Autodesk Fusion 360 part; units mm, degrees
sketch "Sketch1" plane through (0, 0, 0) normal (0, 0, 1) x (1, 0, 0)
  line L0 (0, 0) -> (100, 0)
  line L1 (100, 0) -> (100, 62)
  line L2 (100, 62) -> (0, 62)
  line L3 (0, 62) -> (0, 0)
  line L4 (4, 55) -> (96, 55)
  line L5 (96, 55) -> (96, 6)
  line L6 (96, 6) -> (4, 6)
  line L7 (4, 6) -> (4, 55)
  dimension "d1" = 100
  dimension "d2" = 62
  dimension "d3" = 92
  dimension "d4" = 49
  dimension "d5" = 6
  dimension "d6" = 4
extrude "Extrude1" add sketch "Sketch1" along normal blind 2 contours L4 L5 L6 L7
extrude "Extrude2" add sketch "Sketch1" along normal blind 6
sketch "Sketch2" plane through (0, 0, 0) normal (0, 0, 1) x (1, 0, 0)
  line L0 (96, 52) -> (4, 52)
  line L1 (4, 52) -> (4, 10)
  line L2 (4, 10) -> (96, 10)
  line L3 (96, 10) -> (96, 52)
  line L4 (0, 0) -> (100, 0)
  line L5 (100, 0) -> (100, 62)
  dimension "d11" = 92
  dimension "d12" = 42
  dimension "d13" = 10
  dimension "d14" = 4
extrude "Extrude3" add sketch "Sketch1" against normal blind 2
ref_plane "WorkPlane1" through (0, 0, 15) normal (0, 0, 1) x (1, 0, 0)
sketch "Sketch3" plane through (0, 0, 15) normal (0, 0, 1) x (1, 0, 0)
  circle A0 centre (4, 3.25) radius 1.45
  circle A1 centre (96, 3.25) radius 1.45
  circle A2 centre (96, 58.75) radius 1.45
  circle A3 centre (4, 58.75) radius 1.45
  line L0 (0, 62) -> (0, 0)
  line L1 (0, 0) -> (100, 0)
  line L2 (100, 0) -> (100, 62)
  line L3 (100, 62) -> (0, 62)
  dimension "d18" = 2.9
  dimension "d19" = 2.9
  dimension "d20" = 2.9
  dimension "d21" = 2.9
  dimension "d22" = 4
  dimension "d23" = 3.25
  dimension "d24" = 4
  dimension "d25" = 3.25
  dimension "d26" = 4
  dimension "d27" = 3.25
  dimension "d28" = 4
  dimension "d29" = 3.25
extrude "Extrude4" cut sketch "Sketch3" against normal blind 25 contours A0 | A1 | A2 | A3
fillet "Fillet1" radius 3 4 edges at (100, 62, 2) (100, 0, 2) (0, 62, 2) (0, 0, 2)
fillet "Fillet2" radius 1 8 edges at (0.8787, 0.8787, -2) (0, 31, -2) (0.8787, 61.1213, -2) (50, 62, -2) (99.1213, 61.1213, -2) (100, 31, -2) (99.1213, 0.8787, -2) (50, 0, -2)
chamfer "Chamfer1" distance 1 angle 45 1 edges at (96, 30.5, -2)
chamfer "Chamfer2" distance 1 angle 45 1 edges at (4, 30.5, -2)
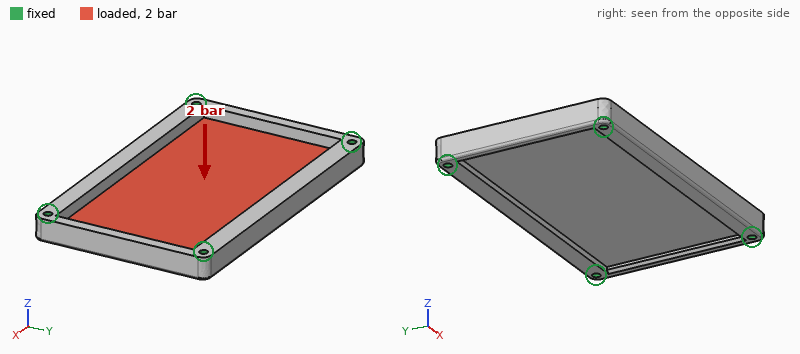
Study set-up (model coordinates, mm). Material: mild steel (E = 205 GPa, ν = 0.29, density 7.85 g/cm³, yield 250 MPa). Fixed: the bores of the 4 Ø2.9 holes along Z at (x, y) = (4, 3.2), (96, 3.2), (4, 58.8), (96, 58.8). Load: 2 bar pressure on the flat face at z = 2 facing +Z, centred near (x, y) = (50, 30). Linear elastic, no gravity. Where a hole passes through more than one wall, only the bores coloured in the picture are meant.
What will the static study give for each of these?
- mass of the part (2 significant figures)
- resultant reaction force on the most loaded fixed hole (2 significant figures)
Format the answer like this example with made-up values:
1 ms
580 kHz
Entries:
170 g
240 N
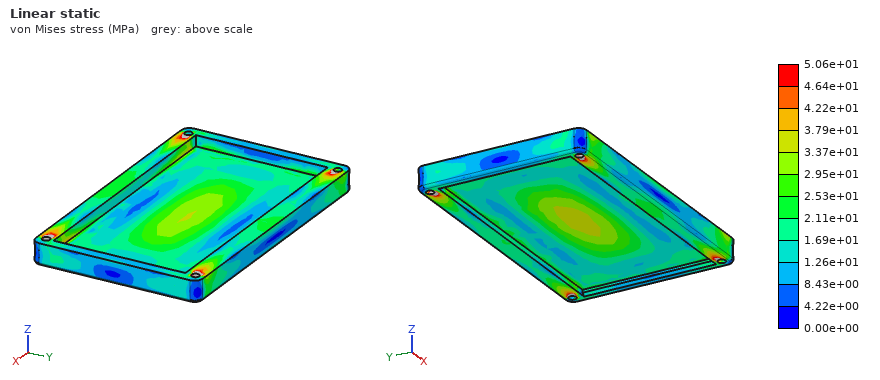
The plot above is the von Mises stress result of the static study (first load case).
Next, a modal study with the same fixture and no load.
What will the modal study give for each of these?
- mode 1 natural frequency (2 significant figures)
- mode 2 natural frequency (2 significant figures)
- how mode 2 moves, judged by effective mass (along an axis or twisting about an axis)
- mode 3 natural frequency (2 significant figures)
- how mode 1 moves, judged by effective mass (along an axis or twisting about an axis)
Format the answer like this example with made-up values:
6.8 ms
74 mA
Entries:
2900 Hz
4300 Hz
twisting about X
5400 Hz
along Z
